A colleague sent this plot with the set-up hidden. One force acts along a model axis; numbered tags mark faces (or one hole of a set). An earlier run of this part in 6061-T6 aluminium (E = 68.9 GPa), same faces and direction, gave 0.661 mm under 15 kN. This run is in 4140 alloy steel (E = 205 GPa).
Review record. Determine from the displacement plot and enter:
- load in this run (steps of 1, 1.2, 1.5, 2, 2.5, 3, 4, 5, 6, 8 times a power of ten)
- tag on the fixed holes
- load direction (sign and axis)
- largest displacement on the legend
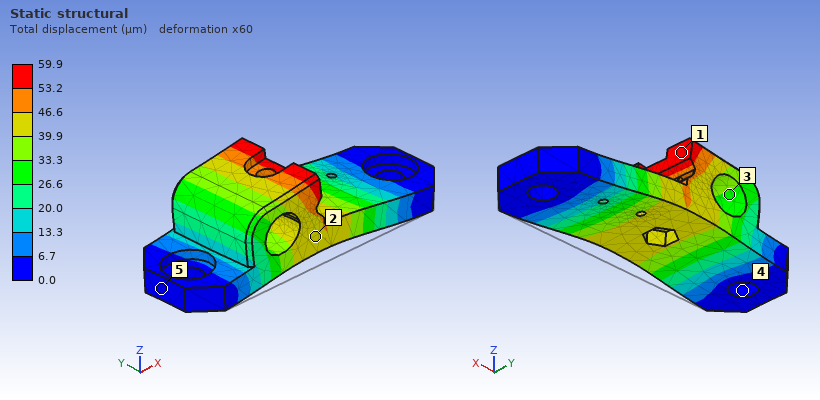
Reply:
4 kN
4
+Z
59.9 µm
